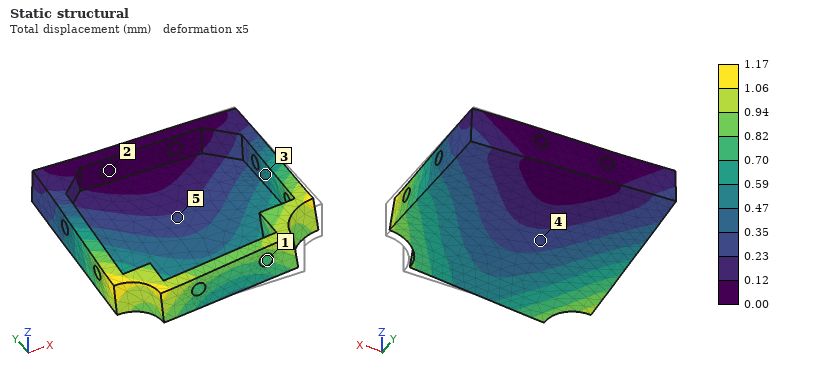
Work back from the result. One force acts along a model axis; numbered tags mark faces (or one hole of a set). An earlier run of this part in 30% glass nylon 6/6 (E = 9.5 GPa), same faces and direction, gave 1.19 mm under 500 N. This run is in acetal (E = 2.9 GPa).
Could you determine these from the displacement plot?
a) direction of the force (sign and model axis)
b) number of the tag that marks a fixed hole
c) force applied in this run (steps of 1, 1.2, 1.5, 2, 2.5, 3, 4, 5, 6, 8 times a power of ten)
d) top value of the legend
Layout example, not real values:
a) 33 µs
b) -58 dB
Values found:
a) -X
b) 2
c) 150 N
d) 1.17 mm
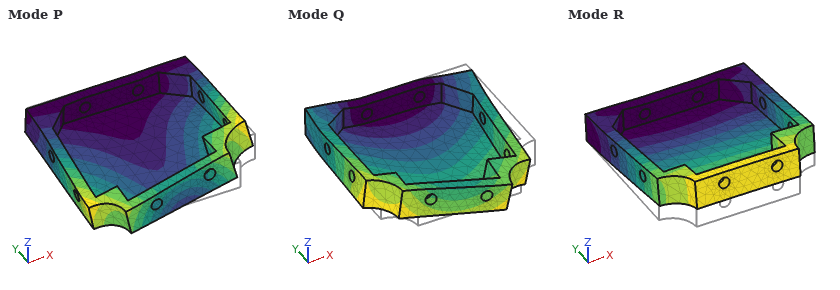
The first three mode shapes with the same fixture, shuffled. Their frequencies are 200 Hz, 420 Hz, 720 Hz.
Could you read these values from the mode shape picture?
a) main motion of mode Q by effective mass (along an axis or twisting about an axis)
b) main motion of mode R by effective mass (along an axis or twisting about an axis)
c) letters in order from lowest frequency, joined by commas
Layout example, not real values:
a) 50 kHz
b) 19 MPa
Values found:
a) along X
b) along Z
c) R, P, Q
